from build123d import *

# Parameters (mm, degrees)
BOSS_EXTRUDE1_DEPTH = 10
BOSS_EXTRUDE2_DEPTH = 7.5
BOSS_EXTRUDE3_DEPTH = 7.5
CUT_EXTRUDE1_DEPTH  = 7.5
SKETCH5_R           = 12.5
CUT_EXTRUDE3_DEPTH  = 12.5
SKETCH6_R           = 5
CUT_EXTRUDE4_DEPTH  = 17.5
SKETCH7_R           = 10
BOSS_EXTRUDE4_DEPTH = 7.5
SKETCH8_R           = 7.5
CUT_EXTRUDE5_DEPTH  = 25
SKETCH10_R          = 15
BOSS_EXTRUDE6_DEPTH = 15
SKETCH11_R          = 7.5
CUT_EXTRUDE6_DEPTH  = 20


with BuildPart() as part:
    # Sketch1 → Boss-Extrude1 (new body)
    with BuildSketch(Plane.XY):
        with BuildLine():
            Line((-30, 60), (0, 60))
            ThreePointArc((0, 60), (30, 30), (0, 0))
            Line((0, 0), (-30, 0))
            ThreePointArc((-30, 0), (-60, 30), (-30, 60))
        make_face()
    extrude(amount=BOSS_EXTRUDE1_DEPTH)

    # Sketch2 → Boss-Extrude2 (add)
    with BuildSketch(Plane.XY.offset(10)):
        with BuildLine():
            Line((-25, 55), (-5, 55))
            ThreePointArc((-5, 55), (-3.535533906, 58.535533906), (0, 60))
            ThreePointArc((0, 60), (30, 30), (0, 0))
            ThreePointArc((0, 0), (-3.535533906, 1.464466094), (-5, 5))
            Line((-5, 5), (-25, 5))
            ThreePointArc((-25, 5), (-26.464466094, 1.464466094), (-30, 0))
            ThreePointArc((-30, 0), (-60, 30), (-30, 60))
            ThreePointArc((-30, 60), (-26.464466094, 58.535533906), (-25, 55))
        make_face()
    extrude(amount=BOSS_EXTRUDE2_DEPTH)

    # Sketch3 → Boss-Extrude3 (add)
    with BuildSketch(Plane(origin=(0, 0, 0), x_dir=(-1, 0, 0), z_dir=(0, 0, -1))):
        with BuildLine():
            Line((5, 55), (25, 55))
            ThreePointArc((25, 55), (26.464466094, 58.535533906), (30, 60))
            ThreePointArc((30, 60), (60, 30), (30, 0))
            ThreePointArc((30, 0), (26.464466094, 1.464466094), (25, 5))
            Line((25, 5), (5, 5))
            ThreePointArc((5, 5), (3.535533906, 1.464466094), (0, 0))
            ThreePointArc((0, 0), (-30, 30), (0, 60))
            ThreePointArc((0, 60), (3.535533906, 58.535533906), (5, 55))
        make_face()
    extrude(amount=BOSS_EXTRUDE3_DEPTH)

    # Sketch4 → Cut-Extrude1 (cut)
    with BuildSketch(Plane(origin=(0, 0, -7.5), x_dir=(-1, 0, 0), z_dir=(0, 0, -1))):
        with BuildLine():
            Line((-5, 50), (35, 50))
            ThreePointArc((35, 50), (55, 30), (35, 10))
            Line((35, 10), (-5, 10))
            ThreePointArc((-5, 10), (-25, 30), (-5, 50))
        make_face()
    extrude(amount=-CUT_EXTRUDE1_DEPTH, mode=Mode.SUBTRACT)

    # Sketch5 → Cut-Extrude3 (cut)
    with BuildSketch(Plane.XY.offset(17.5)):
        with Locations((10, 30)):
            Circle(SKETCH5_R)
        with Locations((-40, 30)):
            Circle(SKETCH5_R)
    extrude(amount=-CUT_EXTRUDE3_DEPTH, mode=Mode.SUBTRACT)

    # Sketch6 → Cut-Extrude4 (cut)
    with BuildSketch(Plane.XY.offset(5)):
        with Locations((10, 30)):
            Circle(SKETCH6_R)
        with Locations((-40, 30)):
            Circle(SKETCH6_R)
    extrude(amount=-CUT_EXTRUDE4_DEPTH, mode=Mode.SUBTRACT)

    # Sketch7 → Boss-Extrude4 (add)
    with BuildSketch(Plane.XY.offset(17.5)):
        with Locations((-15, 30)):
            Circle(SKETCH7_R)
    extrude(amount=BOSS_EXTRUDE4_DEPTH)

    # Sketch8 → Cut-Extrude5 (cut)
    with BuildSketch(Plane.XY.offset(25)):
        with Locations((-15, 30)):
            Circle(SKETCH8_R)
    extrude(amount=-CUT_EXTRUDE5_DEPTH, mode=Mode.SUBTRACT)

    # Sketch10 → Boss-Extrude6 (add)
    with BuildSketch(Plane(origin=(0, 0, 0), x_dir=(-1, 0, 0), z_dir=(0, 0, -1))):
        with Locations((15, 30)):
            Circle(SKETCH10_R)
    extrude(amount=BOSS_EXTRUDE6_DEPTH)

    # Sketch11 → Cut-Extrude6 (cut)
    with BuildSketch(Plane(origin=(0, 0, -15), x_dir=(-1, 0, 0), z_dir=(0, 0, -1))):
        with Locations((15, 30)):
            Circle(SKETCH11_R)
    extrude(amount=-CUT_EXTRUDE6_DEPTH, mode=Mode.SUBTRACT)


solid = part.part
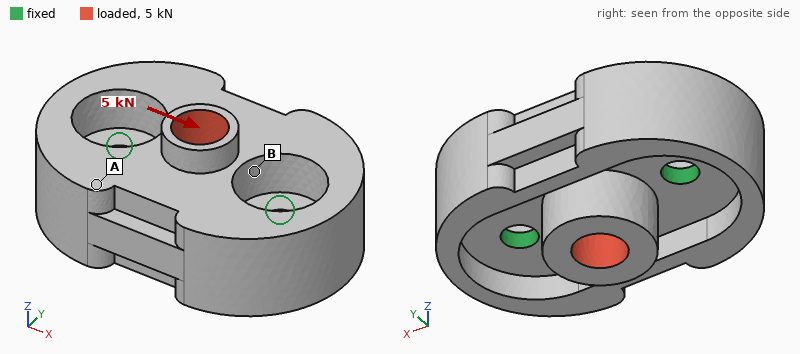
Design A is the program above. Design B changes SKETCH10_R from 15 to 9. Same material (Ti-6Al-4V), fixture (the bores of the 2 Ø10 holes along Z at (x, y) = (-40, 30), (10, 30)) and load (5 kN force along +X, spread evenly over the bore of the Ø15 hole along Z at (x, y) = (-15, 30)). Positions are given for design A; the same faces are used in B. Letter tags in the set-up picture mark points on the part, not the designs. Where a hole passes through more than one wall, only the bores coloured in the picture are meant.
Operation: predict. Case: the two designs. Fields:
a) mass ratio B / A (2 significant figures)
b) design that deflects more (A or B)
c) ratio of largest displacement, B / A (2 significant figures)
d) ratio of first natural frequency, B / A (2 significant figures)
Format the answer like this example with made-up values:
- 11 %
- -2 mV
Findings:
- 0.92
- B
- 3.1
- 1.0
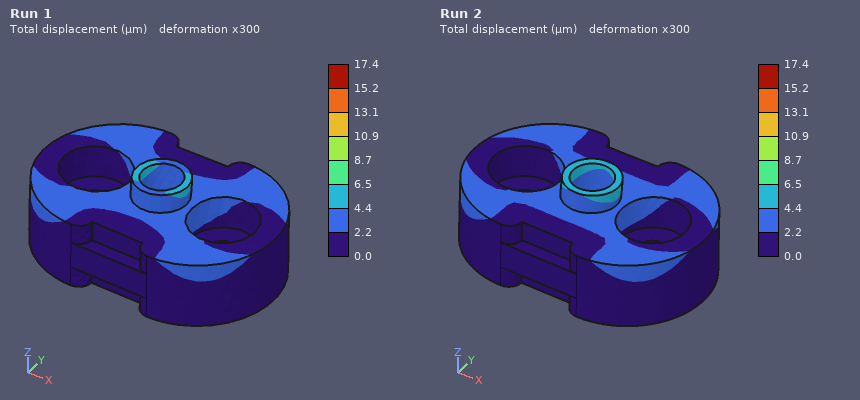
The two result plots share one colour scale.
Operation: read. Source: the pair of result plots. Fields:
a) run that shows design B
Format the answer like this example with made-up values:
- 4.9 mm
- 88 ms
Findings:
- Run 1
